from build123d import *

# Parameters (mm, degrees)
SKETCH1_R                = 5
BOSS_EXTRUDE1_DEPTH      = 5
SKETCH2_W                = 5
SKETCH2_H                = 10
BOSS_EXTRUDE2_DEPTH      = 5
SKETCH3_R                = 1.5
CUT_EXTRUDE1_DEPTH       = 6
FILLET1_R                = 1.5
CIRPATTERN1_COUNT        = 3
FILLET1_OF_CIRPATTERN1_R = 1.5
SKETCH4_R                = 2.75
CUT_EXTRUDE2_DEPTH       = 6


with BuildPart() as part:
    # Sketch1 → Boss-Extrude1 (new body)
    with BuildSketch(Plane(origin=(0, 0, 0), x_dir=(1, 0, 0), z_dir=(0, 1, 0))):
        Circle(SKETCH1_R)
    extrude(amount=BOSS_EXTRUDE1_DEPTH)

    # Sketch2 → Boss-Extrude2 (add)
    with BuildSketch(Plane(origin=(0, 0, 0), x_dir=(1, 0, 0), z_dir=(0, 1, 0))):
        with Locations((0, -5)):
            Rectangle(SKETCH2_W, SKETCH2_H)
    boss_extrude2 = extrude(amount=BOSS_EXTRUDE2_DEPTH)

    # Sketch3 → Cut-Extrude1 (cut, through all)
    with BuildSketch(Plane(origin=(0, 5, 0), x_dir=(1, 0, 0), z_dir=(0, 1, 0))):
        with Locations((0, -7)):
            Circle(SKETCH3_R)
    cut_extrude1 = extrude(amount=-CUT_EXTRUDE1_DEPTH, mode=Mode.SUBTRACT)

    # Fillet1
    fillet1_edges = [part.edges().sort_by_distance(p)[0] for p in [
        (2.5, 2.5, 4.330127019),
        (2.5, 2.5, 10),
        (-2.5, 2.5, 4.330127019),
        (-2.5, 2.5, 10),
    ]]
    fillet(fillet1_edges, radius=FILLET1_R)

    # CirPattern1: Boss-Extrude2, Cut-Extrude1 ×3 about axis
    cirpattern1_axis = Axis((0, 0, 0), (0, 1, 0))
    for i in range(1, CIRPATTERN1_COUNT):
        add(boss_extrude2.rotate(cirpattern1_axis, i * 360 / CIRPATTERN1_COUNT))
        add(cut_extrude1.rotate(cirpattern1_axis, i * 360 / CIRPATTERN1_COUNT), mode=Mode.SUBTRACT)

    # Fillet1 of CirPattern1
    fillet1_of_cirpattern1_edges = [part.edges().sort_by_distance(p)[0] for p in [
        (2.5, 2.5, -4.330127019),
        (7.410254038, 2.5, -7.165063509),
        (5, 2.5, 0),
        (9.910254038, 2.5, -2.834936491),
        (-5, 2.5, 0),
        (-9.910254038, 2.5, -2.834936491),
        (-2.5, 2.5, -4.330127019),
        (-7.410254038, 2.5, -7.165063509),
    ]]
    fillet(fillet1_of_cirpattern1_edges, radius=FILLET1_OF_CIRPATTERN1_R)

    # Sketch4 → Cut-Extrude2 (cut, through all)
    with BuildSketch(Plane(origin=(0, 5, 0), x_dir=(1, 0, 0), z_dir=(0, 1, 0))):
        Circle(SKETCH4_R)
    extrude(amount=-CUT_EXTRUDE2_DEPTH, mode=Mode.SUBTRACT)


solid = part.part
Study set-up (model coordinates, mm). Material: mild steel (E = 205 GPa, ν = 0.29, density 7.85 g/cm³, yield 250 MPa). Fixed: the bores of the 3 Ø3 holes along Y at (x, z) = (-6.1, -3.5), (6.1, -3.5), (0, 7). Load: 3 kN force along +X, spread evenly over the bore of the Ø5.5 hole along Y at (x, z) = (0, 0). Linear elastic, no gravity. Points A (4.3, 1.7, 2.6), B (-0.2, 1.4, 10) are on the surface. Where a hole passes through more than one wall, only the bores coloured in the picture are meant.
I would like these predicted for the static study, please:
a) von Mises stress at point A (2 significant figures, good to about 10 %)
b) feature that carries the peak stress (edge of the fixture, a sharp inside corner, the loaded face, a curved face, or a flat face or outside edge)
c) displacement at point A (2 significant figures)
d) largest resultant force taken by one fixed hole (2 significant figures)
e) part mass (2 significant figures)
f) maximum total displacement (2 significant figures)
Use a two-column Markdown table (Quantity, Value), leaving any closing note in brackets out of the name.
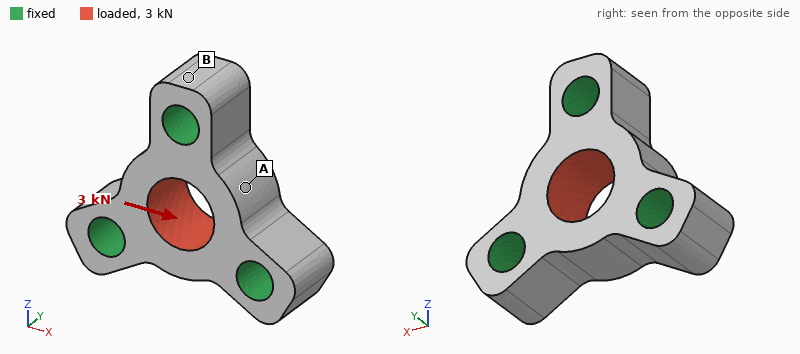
| Quantity | Value |
|---|---|
| von Mises stress at point A | 62 MPa |
| feature that carries the peak stress | edge of the fixture |
| displacement at point A | 2.5 µm |
| largest resultant force taken by one fixed hole | 1.0 kN |
| part mass | 4.3 g |
| maximum total displacement | 2.9 µm |
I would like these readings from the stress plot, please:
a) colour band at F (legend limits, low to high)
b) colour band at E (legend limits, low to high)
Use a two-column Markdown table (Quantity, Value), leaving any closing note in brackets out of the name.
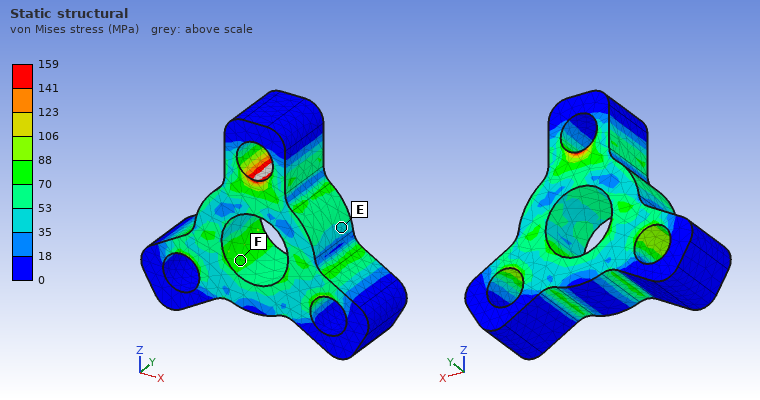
| Quantity | Value |
|---|---|
| colour band at F | 70 to 88 MPa |
| colour band at E | 35 to 53 MPa |
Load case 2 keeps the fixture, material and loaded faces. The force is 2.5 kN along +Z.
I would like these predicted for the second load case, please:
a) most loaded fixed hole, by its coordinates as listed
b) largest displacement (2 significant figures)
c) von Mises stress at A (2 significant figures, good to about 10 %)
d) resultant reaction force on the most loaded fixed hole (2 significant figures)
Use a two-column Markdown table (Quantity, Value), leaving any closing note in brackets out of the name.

| Quantity | Value |
|---|---|
| most loaded fixed hole, by its coordinates as listed | (0, 7) |
| largest displacement | 2.8 µm |
| von Mises stress at A | 28 MPa |
| resultant reaction force on the most loaded fixed hole | 910 N |
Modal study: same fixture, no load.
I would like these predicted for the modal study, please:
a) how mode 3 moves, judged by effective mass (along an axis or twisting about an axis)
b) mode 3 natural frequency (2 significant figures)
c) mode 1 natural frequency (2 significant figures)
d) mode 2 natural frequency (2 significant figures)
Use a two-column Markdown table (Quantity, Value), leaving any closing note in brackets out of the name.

| Quantity | Value |
|---|---|
| how mode 3 moves, judged by effective mass | along Y |
| mode 3 natural frequency | 140 kHz |
| mode 1 natural frequency | 130 kHz |
| mode 2 natural frequency | 130 kHz |
